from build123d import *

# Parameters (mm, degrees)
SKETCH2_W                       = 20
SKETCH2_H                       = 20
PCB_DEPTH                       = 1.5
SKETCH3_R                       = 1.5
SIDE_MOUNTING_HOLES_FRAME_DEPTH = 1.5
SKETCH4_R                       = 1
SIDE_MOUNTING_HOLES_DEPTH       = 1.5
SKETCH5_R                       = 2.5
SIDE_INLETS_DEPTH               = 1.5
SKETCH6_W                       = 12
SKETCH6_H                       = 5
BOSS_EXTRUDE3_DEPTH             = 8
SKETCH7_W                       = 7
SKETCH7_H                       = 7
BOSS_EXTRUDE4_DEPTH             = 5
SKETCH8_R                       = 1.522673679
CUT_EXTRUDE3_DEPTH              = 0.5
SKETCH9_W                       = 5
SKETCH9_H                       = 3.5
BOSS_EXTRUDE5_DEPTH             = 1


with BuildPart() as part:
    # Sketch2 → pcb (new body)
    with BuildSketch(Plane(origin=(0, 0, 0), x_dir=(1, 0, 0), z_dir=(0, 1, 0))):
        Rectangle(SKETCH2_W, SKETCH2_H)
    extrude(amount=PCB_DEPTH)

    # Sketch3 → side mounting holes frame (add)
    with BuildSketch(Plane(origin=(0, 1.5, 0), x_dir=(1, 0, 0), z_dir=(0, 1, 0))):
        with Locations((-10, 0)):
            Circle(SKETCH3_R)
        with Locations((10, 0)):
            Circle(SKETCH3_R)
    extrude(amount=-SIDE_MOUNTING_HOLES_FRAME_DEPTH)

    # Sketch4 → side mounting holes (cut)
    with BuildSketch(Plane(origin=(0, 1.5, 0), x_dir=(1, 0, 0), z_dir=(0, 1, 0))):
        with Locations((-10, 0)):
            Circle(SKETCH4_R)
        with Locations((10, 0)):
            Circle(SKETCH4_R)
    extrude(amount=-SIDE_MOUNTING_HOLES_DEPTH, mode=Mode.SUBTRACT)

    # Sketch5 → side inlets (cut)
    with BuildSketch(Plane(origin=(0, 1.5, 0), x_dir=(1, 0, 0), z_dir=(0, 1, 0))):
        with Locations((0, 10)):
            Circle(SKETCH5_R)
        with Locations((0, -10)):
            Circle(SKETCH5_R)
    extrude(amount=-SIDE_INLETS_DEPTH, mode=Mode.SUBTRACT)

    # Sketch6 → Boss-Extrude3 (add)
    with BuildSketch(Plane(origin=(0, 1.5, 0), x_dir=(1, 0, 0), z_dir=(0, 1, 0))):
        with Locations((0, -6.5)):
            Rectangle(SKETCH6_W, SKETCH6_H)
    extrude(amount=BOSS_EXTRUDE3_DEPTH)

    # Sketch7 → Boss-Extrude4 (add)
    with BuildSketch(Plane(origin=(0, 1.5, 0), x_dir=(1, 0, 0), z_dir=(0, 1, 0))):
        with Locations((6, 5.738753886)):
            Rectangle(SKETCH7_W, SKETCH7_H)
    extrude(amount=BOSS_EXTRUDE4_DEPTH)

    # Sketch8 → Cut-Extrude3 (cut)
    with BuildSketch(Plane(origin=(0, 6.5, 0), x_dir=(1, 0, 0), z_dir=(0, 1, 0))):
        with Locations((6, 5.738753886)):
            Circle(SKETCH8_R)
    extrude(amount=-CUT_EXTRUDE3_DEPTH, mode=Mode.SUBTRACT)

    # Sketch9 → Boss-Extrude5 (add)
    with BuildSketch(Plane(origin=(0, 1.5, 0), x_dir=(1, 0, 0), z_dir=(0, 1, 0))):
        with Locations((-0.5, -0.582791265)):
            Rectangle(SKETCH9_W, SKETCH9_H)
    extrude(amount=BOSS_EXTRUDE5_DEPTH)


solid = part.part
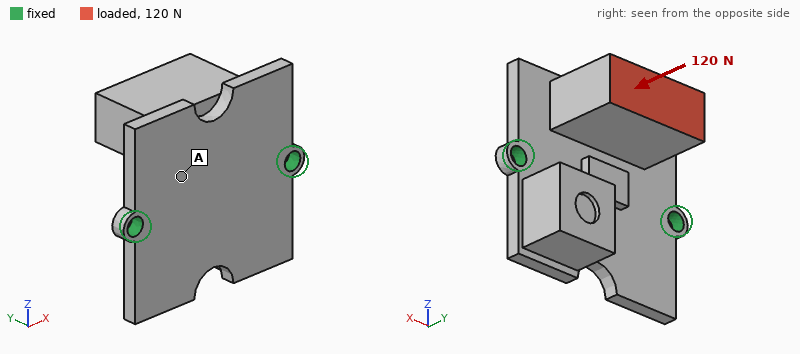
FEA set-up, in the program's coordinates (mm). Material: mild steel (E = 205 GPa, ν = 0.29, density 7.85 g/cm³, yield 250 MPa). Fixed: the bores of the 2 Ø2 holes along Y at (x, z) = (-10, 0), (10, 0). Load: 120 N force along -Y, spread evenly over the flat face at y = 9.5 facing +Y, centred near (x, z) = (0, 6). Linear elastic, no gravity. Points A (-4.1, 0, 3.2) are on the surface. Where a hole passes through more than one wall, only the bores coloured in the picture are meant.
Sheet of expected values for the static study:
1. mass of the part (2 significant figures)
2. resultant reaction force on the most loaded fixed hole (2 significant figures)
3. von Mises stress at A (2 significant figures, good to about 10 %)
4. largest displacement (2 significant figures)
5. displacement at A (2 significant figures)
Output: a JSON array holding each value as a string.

["10 g", "62 N", "48 MPa", "35 µm", "8.3 µm"]
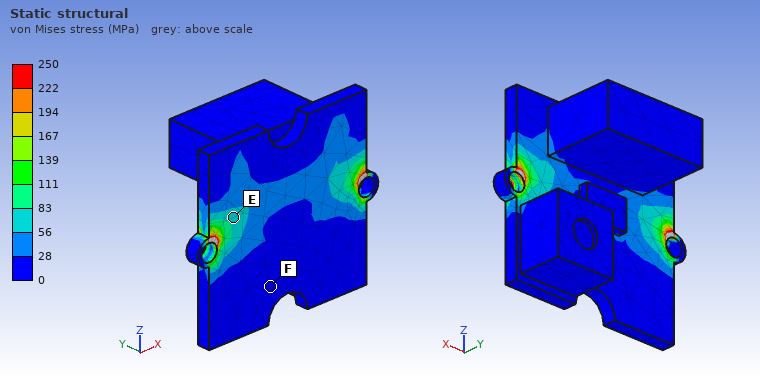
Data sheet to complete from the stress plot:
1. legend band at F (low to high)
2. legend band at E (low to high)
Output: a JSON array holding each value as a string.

["0 to 28 MPa", "56 to 83 MPa"]
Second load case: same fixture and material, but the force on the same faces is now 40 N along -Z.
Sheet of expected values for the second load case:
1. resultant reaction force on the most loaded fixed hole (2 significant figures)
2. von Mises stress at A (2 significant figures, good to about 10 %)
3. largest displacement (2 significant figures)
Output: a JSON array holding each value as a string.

["20 N", "40 MPa", "21 µm"]
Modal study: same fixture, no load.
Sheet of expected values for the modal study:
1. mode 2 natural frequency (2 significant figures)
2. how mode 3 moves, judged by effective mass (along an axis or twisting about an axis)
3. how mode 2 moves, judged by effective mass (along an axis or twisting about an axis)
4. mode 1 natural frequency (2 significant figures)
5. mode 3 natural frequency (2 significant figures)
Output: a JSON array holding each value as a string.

["7500 Hz", "along Y", "along Y", "4200 Hz", "13 kHz"]
